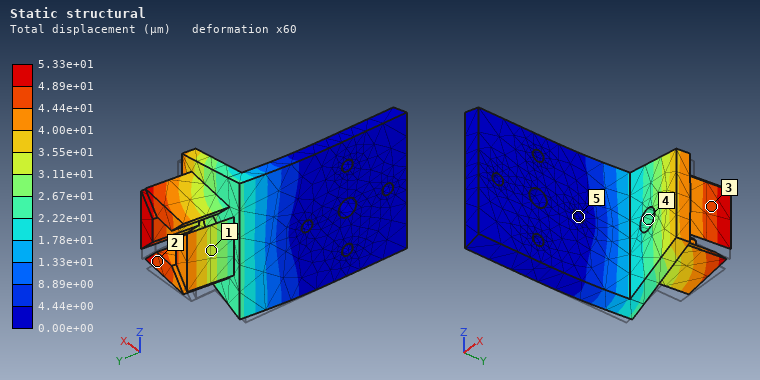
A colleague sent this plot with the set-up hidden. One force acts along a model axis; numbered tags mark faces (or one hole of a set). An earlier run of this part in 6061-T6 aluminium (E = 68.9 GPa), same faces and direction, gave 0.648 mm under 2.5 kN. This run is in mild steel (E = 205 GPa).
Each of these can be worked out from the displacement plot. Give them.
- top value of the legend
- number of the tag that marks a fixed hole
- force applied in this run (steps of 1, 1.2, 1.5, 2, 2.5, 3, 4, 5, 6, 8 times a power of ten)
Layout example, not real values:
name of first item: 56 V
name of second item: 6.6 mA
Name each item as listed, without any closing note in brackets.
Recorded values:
top value of the legend: 5.33e+01 µm
number of the tag that marks a fixed hole: 5
force applied in this run: 600 N
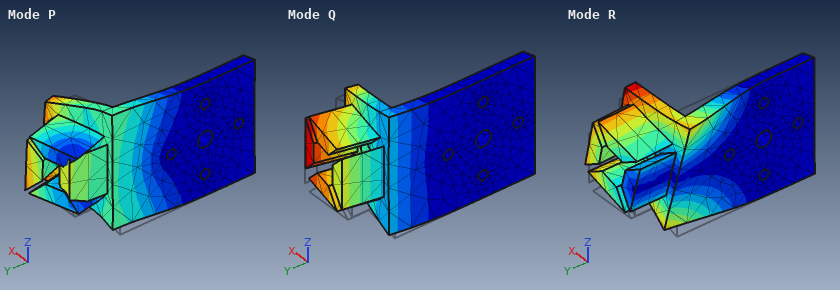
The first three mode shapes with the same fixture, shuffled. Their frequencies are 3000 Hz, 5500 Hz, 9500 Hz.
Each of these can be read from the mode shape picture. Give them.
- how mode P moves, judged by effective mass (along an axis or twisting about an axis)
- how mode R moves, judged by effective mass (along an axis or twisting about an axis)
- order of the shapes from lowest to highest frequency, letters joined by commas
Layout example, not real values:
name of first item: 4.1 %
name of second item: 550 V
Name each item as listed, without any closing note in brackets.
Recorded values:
how mode P moves, judged by effective mass: along X
how mode R moves, judged by effective mass: along Z
order of the shapes from lowest to highest frequency, letters joined by commas: Q, R, P
